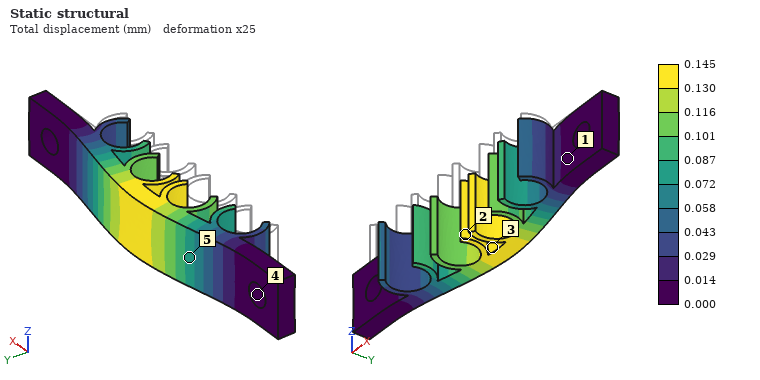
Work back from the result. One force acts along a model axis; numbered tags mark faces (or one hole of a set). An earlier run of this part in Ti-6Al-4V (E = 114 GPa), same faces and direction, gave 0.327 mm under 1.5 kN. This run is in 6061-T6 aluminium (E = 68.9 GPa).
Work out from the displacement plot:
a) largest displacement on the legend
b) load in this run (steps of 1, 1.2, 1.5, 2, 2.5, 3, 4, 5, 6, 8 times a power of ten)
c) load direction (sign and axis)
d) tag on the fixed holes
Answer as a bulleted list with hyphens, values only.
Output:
- 0.145 mm
- 400 N
- +Y
- 4
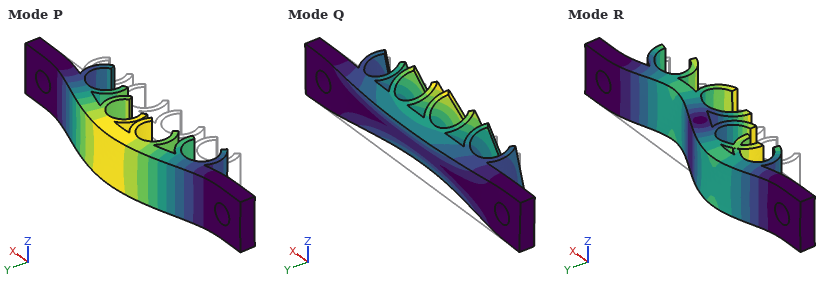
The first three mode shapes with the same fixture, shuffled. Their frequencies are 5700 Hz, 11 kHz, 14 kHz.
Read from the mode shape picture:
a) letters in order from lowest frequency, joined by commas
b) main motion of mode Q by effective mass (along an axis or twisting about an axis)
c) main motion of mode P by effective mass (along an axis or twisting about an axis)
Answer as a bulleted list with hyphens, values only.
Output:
- P, Q, R
- along Z
- along Y
